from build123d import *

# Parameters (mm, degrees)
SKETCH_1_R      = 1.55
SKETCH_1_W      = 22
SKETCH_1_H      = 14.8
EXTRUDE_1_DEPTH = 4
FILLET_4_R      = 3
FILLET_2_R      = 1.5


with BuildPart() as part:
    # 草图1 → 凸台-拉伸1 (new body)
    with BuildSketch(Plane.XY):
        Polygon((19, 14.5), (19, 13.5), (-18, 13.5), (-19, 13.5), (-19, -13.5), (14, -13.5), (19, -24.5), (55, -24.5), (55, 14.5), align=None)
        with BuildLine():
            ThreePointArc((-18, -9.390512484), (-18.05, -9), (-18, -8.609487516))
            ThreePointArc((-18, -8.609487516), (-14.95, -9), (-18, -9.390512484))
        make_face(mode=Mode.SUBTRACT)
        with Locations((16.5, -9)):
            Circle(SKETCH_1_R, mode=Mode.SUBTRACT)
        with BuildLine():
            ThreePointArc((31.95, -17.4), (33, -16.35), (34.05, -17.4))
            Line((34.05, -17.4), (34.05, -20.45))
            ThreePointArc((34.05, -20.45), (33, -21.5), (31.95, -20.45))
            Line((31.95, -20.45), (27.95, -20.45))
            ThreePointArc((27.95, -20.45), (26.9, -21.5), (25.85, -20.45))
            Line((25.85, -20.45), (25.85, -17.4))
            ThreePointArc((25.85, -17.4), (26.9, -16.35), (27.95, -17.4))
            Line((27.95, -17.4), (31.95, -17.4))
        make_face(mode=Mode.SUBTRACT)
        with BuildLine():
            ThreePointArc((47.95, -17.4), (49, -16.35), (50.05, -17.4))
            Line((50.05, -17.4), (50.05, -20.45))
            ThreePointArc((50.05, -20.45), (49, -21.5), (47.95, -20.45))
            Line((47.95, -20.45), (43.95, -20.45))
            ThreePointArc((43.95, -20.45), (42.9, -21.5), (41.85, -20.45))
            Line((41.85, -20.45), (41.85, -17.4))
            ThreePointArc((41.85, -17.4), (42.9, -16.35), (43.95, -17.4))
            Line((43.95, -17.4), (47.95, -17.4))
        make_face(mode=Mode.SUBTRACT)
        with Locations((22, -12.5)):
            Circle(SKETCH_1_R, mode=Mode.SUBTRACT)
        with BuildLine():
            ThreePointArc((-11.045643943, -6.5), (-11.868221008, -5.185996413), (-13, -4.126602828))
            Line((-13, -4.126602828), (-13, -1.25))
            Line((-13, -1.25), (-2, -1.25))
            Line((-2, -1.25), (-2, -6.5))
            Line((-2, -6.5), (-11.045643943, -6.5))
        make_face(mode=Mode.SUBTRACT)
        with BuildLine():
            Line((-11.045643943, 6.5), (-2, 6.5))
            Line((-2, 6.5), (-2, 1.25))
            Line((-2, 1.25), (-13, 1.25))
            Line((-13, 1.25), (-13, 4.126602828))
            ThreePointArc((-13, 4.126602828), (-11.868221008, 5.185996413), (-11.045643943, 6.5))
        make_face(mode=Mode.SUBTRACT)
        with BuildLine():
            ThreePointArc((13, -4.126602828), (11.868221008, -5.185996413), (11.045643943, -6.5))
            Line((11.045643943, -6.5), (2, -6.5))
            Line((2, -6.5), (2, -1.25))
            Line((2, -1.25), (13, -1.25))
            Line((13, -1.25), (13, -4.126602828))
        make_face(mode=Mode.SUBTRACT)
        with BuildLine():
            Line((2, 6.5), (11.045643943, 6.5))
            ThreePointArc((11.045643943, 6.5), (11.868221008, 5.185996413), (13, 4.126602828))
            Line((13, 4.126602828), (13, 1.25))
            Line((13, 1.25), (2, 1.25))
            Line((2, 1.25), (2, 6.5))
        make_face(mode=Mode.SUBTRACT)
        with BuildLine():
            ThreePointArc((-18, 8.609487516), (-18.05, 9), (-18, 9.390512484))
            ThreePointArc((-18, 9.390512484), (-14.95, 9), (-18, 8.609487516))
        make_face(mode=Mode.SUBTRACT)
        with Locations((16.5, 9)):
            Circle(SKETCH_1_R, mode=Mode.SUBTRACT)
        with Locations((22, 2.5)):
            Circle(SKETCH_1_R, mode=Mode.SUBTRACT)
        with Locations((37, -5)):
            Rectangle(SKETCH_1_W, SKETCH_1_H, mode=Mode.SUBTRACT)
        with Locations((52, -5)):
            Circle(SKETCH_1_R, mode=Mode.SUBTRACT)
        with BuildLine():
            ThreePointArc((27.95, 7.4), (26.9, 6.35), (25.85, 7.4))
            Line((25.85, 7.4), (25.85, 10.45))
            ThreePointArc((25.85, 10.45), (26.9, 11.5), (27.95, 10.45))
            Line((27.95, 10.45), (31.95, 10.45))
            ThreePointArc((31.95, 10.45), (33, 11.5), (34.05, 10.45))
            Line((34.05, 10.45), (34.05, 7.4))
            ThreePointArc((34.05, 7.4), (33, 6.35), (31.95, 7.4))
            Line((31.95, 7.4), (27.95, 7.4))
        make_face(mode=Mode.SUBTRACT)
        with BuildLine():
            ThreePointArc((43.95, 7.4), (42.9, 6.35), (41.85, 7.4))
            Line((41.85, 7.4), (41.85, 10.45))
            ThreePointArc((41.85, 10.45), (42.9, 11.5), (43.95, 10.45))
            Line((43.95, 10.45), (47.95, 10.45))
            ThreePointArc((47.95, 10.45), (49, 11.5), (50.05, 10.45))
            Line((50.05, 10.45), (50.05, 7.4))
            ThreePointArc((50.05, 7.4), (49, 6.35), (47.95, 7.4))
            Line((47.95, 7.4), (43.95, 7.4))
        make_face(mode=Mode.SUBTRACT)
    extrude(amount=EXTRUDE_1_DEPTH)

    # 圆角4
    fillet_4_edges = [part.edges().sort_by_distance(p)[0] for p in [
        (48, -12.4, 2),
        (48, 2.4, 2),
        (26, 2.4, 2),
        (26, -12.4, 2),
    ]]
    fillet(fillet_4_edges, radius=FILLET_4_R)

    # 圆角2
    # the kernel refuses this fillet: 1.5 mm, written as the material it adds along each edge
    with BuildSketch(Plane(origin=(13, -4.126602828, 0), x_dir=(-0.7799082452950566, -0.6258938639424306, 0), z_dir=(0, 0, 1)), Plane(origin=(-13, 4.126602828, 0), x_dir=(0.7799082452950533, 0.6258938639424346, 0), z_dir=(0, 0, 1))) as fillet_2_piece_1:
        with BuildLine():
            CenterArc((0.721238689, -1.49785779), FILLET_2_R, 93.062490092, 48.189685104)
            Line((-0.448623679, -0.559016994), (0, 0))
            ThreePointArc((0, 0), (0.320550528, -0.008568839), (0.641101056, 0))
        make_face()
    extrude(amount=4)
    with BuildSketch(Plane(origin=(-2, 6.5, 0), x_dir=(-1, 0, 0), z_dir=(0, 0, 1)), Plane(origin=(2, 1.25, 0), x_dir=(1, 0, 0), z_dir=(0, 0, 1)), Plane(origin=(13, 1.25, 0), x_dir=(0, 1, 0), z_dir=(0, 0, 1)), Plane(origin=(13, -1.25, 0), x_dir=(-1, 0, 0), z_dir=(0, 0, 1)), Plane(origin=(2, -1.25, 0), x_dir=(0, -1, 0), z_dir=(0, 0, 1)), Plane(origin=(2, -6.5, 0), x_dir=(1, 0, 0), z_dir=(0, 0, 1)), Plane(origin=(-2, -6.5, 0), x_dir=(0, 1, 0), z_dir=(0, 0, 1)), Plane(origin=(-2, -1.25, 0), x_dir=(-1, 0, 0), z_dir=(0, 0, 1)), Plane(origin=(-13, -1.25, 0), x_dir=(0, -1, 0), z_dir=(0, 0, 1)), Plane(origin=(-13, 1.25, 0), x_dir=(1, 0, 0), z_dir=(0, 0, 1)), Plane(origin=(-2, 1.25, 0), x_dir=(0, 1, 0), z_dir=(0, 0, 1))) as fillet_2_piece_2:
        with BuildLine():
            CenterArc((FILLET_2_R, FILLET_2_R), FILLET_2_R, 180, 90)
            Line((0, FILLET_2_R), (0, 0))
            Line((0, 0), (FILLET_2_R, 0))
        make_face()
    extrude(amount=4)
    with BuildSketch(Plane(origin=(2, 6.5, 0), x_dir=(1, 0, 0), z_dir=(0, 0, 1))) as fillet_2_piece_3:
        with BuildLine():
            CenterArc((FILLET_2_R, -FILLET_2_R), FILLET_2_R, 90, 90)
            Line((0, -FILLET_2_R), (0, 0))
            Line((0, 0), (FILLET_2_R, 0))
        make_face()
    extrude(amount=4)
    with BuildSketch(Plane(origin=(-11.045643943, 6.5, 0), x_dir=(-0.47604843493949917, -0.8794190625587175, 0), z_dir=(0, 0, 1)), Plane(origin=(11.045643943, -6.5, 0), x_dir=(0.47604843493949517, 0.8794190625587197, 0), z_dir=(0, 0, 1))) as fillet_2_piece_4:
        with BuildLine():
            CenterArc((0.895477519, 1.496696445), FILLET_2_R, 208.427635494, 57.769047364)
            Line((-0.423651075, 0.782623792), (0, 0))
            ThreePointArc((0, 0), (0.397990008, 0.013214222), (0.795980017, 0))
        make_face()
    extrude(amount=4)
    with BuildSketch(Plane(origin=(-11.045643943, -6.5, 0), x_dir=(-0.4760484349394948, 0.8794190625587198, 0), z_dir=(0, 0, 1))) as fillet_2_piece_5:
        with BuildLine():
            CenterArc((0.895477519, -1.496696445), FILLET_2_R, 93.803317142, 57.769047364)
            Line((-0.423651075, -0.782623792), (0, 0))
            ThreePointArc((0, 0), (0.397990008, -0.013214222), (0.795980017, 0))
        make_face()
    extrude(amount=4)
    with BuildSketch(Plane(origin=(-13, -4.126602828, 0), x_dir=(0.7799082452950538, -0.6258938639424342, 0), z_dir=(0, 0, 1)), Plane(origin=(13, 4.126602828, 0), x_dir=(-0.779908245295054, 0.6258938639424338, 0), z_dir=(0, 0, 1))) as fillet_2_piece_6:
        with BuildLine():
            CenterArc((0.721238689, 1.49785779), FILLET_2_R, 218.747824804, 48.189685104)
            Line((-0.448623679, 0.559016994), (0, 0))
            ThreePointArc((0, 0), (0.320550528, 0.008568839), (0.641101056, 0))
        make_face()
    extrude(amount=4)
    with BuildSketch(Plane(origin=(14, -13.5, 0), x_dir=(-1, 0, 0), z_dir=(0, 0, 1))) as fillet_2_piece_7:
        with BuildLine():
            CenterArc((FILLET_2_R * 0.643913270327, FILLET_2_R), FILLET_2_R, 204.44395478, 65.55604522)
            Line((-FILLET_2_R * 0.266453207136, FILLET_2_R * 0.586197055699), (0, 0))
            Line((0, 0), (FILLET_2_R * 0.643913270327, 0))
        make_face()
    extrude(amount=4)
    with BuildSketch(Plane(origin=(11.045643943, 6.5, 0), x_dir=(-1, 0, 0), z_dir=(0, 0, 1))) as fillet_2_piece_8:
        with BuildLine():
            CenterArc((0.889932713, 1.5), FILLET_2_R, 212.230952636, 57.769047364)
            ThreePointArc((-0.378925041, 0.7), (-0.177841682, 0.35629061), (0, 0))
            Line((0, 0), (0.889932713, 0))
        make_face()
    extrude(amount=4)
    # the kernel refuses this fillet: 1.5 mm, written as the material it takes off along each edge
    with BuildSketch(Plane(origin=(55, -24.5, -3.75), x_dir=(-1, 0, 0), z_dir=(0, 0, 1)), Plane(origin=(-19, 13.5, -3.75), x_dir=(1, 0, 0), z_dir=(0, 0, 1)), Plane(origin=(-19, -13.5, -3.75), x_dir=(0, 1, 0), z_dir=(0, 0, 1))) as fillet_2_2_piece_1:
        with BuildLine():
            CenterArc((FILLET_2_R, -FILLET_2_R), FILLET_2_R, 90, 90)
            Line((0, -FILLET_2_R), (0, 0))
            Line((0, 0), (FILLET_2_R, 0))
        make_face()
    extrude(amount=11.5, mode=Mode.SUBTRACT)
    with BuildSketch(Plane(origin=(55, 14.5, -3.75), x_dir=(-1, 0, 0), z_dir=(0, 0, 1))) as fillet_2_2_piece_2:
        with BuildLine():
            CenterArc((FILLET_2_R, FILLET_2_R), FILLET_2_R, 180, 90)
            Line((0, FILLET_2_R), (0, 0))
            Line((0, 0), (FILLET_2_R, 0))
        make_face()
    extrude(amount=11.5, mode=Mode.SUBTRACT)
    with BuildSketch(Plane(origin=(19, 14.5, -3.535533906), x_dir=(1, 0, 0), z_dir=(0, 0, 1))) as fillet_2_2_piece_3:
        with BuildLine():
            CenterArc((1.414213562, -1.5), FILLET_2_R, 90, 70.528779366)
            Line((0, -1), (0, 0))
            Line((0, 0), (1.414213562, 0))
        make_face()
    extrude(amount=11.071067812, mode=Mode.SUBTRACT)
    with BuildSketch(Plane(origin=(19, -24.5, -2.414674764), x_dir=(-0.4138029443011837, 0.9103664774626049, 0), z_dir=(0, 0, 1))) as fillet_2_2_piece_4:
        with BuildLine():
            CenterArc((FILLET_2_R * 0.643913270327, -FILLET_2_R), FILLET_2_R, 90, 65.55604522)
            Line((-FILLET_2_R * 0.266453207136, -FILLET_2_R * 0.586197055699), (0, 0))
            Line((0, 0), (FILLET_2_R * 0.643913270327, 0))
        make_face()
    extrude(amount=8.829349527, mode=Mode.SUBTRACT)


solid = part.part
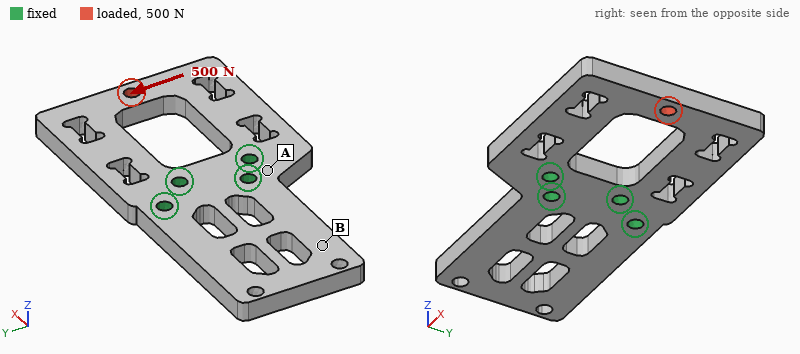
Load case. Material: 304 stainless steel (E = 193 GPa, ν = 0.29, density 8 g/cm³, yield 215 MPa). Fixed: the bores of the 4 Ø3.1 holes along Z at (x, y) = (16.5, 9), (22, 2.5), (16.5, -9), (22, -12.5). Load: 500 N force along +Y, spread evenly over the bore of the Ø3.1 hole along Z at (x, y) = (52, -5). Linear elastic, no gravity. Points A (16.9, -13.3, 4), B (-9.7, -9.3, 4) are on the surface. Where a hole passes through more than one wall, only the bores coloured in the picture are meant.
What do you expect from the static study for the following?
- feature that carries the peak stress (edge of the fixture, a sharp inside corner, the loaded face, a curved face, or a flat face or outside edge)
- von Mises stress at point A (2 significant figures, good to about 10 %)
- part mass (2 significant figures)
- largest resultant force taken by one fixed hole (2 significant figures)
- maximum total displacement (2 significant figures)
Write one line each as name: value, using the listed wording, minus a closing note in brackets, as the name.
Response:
feature that carries the peak stress: a curved face
von Mises stress at point A: 23 MPa
part mass: 56 g
largest resultant force taken by one fixed hole: 640 N
maximum total displacement: 22 µm
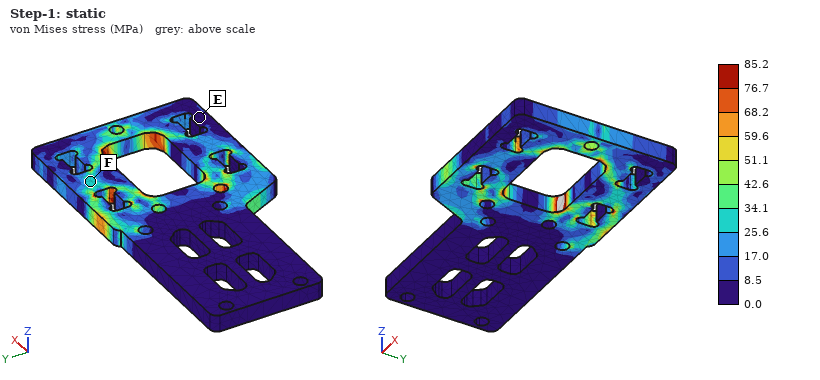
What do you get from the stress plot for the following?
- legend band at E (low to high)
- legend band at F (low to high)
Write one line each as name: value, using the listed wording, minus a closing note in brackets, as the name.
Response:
legend band at E: 0.0 to 8.5 MPa
legend band at F: 25.6 to 34.1 MPa
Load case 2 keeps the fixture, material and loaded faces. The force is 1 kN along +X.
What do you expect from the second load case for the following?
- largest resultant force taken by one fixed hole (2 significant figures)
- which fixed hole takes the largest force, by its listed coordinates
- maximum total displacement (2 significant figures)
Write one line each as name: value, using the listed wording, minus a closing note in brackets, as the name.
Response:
largest resultant force taken by one fixed hole: 560 N
which fixed hole takes the largest force, by its listed coordinates: (22, -12.5)
maximum total displacement: 9.5 µm
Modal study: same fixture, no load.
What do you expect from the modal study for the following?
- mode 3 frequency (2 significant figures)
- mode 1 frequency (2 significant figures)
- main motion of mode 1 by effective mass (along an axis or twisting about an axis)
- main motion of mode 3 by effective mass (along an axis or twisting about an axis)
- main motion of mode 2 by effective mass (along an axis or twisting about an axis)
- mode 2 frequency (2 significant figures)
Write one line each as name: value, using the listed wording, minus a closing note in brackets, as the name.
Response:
mode 3 frequency: 4100 Hz
mode 1 frequency: 2200 Hz
main motion of mode 1 by effective mass: along Z
main motion of mode 3 by effective mass: twisting about X
main motion of mode 2 by effective mass: along Z
mode 2 frequency: 2400 Hz
